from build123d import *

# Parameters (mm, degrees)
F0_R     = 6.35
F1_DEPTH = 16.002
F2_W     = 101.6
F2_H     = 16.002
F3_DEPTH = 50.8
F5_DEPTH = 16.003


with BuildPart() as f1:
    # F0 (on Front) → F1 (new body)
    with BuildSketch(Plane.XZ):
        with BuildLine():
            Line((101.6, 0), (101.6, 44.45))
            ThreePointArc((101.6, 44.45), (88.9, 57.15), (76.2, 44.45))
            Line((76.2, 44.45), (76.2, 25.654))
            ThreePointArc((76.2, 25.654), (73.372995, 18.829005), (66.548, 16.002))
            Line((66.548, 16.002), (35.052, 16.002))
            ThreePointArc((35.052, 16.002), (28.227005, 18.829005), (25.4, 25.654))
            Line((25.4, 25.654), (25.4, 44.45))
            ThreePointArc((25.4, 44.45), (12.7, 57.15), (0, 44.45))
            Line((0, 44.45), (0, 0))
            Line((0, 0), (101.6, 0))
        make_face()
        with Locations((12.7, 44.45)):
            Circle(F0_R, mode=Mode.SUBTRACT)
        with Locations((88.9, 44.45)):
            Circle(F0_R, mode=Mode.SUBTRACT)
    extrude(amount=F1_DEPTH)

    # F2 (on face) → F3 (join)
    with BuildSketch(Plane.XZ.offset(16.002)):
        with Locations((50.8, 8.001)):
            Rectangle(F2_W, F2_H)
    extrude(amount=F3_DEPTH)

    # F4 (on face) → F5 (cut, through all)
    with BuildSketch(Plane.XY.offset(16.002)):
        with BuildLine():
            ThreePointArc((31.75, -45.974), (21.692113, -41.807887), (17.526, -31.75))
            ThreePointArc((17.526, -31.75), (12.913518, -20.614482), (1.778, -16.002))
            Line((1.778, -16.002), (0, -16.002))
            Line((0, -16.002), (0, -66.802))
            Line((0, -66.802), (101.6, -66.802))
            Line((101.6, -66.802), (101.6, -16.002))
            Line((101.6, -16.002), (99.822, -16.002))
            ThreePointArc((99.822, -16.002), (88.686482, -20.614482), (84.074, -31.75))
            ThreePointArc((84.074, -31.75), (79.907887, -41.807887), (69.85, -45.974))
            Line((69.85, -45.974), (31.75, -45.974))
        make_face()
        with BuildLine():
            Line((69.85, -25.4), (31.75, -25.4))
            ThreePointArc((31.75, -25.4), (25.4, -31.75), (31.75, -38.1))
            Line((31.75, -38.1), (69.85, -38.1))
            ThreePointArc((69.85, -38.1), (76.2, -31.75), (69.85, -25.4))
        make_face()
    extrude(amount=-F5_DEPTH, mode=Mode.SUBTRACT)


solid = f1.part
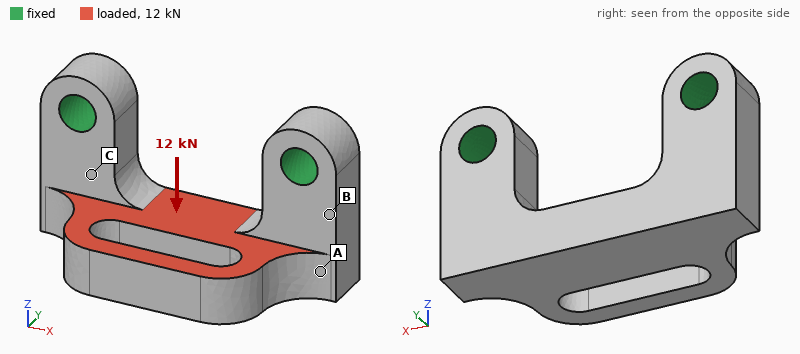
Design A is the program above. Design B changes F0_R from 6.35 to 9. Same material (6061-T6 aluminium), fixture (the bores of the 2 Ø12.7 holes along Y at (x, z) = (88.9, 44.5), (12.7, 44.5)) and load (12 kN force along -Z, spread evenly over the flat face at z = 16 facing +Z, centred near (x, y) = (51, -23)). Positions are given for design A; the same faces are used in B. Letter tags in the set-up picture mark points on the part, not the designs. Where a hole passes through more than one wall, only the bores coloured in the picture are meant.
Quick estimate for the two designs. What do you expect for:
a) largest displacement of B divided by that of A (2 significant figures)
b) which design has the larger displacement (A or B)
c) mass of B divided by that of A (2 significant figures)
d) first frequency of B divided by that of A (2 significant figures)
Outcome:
0.92
A
0.95
1.1
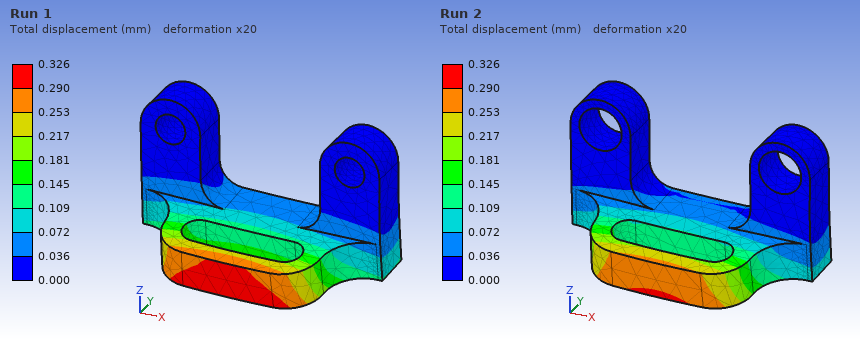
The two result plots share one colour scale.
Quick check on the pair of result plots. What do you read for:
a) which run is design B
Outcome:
Run 2
